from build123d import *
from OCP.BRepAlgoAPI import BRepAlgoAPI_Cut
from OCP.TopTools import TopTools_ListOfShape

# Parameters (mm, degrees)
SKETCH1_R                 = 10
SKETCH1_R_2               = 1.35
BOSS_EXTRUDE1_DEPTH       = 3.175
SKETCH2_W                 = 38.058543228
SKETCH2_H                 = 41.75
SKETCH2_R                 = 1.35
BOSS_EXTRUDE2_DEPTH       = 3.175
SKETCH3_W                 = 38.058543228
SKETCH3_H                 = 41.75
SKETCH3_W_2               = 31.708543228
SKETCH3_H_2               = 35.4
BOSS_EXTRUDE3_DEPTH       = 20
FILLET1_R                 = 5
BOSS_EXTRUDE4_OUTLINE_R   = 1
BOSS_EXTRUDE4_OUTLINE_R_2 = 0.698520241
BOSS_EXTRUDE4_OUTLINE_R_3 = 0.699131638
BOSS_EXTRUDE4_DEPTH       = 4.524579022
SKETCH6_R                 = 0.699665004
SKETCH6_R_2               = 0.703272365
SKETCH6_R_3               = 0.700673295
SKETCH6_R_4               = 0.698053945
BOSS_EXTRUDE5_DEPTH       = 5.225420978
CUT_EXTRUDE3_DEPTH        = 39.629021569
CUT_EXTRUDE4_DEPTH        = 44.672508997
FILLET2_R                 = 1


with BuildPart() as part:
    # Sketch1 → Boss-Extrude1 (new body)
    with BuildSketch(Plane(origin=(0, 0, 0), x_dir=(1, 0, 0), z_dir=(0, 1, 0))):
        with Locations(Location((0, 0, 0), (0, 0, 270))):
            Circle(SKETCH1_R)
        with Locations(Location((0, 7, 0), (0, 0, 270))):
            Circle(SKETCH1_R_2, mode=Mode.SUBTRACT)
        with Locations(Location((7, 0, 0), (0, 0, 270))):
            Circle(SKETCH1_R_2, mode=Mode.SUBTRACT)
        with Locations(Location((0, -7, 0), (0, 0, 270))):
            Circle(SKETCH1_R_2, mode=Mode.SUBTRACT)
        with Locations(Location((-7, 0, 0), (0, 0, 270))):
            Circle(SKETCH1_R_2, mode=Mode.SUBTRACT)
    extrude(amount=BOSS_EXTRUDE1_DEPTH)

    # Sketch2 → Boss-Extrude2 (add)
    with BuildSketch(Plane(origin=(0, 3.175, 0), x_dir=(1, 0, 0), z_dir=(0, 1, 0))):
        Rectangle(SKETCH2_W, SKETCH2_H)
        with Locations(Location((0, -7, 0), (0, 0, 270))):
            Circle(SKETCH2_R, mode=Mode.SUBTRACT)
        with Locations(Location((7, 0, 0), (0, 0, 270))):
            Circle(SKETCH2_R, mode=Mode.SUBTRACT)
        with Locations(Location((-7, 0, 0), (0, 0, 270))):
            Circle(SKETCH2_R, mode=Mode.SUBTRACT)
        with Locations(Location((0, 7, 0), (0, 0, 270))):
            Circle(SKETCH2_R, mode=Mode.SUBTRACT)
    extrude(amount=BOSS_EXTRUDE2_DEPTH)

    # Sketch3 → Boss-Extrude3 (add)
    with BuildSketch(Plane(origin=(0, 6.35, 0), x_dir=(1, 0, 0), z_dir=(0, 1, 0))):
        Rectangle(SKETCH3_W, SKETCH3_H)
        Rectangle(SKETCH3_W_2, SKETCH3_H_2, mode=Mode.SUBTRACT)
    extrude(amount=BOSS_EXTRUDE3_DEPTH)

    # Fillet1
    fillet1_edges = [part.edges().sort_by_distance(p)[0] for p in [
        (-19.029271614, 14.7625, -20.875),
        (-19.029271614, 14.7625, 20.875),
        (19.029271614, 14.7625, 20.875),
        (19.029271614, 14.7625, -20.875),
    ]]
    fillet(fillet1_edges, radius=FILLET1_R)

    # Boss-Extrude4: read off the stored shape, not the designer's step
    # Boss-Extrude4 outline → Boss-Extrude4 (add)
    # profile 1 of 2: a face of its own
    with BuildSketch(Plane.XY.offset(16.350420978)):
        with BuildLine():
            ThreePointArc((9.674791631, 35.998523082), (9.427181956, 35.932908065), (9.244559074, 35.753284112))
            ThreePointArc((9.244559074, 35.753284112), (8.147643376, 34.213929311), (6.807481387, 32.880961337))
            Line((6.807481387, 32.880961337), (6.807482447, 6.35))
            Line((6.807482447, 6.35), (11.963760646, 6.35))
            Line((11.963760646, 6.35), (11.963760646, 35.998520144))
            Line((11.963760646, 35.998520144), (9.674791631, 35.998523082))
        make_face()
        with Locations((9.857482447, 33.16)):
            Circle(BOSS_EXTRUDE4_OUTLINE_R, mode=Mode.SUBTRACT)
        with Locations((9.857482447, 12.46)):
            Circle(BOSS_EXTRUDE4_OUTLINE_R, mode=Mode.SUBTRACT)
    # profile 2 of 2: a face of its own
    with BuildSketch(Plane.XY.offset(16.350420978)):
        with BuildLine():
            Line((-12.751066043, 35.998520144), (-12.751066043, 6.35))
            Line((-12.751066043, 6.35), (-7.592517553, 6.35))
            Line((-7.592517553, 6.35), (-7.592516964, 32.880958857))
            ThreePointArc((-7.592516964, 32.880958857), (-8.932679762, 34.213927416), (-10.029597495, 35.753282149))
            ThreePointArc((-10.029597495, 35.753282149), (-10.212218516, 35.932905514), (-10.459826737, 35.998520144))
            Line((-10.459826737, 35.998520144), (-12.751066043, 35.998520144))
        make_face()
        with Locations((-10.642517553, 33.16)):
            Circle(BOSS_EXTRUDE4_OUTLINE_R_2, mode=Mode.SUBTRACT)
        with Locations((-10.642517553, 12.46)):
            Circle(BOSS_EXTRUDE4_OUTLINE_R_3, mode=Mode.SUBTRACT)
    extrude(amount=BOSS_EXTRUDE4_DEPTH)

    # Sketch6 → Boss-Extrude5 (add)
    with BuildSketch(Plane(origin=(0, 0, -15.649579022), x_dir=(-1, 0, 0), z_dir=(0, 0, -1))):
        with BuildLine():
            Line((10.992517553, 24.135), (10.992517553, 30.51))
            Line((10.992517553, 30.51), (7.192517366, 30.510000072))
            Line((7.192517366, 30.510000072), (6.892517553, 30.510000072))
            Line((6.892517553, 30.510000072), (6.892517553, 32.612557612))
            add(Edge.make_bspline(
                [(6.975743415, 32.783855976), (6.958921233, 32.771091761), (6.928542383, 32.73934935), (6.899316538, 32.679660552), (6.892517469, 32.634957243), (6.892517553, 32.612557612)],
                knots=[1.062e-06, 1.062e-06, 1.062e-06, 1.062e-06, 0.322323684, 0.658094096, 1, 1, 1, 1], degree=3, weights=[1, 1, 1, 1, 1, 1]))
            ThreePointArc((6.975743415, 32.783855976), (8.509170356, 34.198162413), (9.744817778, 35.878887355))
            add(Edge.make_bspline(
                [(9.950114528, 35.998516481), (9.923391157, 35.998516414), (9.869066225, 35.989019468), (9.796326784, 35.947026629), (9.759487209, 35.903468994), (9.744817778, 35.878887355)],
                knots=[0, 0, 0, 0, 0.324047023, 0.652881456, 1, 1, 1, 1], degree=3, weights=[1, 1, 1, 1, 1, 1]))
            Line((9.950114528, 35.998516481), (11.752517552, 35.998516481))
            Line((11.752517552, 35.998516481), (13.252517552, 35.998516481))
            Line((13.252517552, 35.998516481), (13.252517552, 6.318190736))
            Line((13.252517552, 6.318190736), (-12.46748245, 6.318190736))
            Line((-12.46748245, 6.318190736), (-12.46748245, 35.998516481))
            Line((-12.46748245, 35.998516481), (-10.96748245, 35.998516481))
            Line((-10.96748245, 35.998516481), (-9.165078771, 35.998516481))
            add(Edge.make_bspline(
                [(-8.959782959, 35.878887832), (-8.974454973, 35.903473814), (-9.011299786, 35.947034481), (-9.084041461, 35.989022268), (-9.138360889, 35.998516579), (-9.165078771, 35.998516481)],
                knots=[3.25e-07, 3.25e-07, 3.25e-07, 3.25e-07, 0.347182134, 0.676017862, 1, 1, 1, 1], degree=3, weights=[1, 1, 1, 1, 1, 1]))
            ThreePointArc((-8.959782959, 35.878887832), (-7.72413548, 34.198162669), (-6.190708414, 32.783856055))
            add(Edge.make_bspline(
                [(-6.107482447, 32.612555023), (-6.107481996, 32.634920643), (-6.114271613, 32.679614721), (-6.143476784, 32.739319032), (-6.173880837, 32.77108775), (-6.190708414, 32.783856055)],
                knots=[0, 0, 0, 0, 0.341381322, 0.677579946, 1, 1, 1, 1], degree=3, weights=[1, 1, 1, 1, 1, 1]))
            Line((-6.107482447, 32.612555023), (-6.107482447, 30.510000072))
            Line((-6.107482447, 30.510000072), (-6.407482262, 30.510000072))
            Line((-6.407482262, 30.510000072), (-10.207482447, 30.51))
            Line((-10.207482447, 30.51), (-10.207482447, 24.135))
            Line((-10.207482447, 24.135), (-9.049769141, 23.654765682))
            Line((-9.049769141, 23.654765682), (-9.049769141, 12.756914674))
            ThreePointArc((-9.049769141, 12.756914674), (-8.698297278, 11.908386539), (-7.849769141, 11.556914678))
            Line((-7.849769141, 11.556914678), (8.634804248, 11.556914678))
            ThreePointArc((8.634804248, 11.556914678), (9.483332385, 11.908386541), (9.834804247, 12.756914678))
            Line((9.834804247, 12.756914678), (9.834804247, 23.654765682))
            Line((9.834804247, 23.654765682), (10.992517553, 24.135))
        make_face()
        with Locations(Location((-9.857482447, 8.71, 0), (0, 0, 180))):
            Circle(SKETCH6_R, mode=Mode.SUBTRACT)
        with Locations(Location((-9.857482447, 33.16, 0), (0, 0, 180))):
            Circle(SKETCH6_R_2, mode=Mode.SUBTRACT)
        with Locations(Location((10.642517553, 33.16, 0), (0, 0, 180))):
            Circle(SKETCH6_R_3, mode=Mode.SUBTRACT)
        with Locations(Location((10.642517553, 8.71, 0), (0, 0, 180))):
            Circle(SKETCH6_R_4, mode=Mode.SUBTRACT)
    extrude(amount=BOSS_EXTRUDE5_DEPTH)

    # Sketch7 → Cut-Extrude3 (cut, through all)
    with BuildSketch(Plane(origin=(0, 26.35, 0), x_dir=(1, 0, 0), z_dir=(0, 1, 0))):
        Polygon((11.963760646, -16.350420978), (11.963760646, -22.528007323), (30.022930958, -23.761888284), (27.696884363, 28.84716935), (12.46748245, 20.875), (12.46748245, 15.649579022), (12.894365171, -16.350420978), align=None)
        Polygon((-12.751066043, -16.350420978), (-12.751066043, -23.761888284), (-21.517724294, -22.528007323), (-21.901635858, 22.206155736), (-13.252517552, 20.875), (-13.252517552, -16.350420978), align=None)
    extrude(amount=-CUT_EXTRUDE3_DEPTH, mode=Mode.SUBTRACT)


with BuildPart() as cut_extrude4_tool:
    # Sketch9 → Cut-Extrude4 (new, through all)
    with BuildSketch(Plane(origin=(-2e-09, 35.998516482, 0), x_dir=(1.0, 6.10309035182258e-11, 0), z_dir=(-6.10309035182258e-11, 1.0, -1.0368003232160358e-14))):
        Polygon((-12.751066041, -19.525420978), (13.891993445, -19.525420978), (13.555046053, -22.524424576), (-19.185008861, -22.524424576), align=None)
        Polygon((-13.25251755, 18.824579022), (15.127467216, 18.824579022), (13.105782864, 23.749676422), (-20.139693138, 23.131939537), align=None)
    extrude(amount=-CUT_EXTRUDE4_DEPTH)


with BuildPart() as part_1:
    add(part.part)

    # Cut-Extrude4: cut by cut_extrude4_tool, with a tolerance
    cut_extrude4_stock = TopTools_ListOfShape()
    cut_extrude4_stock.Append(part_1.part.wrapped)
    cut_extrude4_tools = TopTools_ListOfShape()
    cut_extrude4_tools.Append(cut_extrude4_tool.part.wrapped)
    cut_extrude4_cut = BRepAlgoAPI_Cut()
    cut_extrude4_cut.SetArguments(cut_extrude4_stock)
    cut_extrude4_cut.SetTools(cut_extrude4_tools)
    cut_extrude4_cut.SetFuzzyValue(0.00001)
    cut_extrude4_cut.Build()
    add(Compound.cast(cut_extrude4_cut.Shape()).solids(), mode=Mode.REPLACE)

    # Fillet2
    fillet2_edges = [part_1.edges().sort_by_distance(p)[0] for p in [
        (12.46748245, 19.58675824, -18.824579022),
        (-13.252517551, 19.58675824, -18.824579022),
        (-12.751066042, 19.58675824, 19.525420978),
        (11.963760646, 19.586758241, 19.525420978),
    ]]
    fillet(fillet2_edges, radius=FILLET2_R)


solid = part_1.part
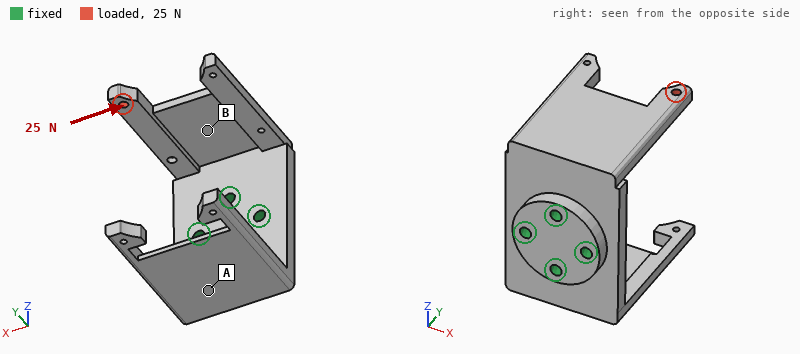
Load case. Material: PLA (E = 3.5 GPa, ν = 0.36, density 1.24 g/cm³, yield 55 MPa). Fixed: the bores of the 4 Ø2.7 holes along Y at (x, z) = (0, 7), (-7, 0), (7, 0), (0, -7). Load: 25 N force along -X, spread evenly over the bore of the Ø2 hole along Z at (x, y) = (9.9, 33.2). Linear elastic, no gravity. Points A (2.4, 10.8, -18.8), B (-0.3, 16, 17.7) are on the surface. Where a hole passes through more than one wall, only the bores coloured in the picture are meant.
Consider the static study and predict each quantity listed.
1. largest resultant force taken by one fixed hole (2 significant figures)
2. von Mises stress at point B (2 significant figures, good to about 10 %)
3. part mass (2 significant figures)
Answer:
26 N
4.3 MPa
8.3 g
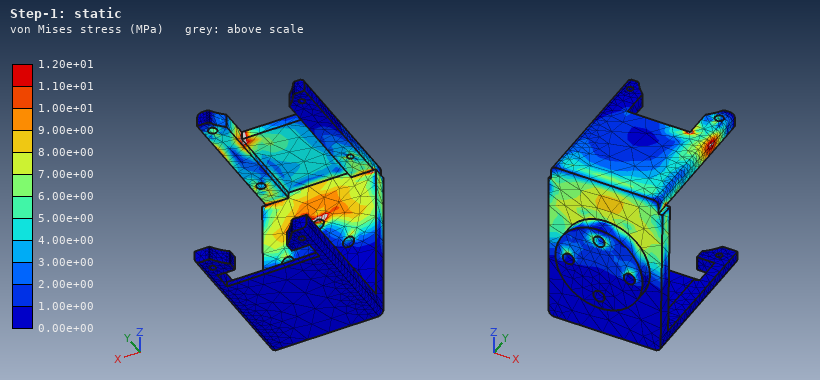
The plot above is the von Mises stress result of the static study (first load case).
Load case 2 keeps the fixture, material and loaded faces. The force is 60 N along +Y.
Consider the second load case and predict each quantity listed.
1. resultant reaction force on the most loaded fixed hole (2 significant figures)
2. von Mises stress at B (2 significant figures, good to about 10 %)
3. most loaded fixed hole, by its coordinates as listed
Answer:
81 N
1.5 MPa
(0, 7)
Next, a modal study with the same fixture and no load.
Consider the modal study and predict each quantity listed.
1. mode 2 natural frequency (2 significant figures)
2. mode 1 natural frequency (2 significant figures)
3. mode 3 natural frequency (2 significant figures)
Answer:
840 Hz
780 Hz
1100 Hz
